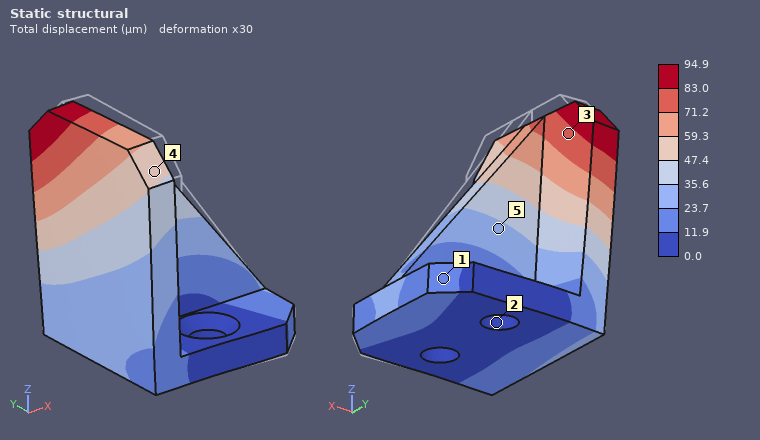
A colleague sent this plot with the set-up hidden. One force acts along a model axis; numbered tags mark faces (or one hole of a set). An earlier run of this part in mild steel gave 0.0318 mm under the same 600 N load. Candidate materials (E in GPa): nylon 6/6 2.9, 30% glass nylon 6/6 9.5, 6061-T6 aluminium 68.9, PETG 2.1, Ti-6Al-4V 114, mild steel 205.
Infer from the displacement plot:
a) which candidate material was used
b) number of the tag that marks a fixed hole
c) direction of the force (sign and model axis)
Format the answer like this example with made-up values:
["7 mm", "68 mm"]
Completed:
["6061-T6 aluminium", "2", "-X"]
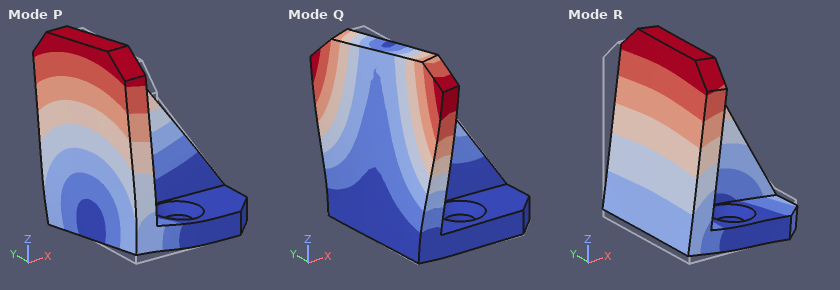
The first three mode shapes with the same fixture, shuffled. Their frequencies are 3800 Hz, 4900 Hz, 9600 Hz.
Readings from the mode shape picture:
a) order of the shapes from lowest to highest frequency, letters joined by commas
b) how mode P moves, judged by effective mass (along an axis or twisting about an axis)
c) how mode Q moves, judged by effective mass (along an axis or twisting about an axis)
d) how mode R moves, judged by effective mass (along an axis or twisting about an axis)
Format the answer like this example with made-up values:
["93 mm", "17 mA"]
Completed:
["R, P, Q", "along Y", "twisting about Z", "along X"]
